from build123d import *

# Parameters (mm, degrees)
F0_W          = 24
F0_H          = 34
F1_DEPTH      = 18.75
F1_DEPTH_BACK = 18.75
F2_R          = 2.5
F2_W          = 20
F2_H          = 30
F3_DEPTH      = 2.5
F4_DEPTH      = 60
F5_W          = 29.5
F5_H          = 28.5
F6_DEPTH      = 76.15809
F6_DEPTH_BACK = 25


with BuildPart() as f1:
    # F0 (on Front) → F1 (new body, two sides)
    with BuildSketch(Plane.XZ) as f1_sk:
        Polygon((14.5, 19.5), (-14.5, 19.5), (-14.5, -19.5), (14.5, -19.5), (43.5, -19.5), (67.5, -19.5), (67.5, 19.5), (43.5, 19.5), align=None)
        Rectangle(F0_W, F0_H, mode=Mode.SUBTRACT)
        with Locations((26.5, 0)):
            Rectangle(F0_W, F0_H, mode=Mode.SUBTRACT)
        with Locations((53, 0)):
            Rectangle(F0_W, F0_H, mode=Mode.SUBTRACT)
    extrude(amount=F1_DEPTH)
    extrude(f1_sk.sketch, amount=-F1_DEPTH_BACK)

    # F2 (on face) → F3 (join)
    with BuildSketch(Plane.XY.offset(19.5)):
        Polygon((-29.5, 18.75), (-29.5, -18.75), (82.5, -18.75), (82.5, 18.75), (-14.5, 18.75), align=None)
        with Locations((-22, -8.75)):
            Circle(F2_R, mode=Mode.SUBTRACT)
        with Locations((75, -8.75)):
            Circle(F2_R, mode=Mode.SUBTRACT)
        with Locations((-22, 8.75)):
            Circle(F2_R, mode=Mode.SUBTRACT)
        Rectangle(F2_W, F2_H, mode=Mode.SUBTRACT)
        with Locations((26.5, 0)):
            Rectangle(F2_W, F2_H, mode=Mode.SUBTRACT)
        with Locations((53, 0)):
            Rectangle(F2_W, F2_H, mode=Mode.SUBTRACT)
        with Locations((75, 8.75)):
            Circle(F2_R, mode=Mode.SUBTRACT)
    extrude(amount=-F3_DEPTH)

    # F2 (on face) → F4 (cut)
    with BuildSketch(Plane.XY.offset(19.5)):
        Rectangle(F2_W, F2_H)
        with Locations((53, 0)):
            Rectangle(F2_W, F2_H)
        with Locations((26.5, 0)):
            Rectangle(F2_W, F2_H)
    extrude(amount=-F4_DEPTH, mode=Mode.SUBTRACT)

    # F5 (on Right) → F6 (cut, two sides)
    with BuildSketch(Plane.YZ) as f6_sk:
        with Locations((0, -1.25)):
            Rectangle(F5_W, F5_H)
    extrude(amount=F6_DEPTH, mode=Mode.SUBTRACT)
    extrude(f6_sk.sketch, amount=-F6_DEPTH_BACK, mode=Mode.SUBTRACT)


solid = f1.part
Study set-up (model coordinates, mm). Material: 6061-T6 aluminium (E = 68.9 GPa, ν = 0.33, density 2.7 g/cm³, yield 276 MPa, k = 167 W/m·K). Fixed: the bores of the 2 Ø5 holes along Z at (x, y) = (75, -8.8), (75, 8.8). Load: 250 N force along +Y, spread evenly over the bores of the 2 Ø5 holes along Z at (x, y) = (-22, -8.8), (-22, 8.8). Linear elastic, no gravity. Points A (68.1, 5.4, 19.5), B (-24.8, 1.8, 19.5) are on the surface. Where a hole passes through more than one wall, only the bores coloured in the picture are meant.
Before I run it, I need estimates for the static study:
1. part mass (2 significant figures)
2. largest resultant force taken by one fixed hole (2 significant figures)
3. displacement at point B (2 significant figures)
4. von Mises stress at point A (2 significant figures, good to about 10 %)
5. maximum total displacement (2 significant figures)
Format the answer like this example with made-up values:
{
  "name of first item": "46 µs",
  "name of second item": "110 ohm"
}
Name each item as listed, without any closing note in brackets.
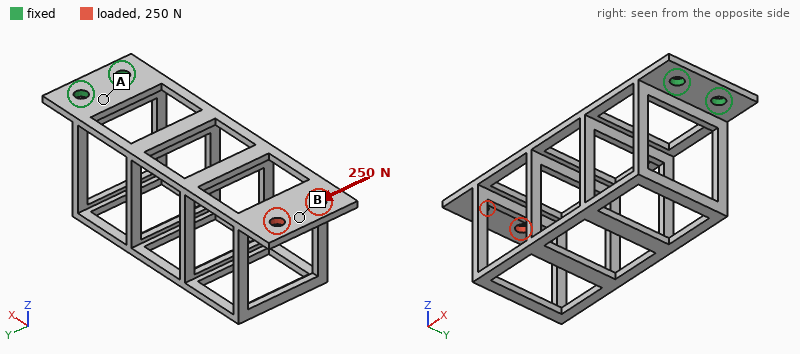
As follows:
{
  "part mass": "36 g",
  "largest resultant force taken by one fixed hole": "1.1 kN",
  "displacement at point B": "0.98 mm",
  "von Mises stress at point A": "37 MPa",
  "maximum total displacement": "1.0 mm"
}
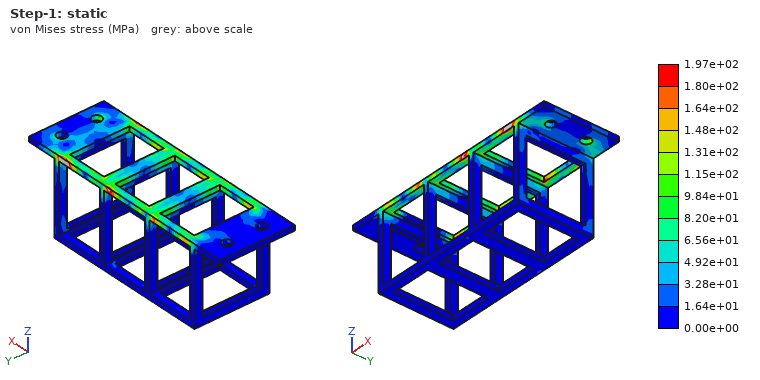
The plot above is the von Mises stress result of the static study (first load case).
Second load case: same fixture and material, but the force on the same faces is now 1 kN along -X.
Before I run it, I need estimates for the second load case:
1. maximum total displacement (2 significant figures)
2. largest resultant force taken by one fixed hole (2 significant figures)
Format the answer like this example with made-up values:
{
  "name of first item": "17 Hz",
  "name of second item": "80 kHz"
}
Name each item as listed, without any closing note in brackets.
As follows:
{
  "maximum total displacement": "0.13 mm",
  "largest resultant force taken by one fixed hole": "530 N"
}
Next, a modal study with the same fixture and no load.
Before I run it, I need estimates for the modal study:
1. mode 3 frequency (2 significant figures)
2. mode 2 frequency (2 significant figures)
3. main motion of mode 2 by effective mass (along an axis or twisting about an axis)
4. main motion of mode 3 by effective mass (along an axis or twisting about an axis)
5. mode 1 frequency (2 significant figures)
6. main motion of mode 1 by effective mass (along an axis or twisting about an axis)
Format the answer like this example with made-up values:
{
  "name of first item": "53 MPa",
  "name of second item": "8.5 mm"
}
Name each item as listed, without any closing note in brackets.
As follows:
{
  "mode 3 frequency": "860 Hz",
  "mode 2 frequency": "570 Hz",
  "main motion of mode 2 by effective mass": "along Y",
  "main motion of mode 3 by effective mass": "along Y",
  "mode 1 frequency": "160 Hz",
  "main motion of mode 1 by effective mass": "along Z"
}
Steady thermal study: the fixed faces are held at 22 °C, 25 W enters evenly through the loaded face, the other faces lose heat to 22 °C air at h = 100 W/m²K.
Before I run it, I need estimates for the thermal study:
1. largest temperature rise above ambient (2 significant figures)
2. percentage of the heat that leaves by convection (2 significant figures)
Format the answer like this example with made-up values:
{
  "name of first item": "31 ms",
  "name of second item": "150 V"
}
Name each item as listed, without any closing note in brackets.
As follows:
{
  "largest temperature rise above ambient": "77 K",
  "percentage of the heat that leaves by convection": "98 %"
}
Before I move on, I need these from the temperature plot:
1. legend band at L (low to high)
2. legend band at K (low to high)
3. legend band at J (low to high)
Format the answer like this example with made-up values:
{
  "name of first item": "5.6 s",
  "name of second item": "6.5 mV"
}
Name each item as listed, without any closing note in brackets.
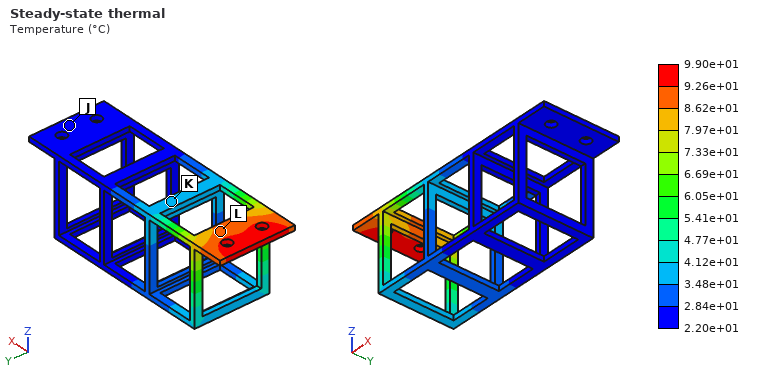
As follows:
{
  "legend band at L": "8.62e+01 to 9.26e+01 °C",
  "legend band at K": "3.48e+01 to 4.12e+01 °C",
  "legend band at J": "2.20e+01 to 2.84e+01 °C"
}
